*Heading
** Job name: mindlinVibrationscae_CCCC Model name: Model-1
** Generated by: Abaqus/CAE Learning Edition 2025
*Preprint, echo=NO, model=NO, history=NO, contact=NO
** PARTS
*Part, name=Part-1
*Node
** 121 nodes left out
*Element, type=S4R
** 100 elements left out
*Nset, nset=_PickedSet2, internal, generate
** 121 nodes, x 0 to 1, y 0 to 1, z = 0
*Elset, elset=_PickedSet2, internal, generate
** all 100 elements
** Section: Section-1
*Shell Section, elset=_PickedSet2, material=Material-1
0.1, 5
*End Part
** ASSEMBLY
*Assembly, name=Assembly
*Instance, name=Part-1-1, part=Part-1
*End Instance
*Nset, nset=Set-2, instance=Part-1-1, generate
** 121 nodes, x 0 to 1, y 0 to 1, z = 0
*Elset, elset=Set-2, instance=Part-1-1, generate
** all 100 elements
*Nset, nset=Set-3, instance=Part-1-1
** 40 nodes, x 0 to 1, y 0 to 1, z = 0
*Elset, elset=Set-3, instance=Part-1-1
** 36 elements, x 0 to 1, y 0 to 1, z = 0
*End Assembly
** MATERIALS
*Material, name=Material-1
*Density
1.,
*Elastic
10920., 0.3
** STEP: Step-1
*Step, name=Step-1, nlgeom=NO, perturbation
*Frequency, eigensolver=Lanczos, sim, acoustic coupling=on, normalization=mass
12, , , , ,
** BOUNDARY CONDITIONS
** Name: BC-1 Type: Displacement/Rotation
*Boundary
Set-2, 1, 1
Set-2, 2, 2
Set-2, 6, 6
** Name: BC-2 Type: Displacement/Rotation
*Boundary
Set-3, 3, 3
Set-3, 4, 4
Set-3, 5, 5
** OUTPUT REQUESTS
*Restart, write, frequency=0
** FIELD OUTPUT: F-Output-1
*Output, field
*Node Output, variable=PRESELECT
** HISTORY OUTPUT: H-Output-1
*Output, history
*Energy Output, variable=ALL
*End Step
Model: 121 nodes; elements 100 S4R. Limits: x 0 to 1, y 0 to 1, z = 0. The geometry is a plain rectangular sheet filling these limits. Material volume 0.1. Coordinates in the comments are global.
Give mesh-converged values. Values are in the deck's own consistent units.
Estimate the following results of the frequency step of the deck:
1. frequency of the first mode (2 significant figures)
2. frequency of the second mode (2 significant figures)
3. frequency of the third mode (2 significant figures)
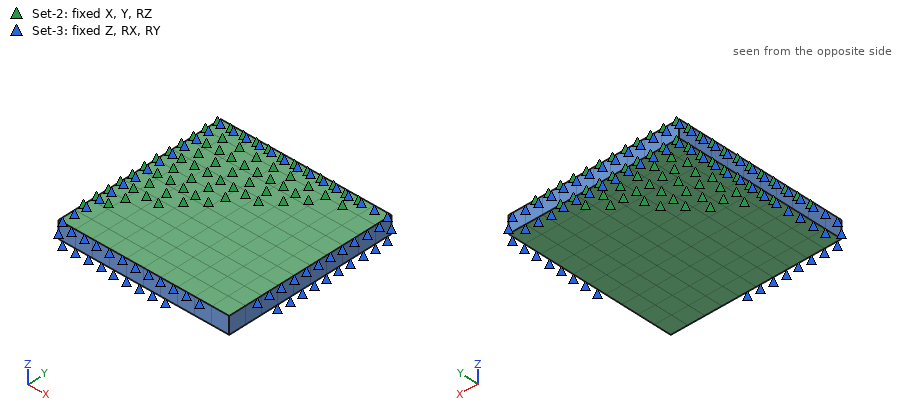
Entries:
17 cycles per unit time
32 cycles per unit time
32 cycles per unit time
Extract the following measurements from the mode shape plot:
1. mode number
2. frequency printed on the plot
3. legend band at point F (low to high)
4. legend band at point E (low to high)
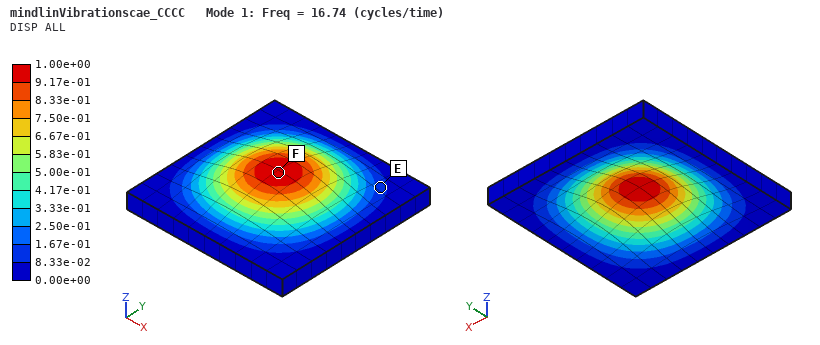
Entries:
1
16.74
9.17e-01 to 1.00e+00
8.33e-02 to 1.67e-01
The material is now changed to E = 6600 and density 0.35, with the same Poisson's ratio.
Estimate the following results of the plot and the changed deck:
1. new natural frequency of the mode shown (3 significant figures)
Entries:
22.0
